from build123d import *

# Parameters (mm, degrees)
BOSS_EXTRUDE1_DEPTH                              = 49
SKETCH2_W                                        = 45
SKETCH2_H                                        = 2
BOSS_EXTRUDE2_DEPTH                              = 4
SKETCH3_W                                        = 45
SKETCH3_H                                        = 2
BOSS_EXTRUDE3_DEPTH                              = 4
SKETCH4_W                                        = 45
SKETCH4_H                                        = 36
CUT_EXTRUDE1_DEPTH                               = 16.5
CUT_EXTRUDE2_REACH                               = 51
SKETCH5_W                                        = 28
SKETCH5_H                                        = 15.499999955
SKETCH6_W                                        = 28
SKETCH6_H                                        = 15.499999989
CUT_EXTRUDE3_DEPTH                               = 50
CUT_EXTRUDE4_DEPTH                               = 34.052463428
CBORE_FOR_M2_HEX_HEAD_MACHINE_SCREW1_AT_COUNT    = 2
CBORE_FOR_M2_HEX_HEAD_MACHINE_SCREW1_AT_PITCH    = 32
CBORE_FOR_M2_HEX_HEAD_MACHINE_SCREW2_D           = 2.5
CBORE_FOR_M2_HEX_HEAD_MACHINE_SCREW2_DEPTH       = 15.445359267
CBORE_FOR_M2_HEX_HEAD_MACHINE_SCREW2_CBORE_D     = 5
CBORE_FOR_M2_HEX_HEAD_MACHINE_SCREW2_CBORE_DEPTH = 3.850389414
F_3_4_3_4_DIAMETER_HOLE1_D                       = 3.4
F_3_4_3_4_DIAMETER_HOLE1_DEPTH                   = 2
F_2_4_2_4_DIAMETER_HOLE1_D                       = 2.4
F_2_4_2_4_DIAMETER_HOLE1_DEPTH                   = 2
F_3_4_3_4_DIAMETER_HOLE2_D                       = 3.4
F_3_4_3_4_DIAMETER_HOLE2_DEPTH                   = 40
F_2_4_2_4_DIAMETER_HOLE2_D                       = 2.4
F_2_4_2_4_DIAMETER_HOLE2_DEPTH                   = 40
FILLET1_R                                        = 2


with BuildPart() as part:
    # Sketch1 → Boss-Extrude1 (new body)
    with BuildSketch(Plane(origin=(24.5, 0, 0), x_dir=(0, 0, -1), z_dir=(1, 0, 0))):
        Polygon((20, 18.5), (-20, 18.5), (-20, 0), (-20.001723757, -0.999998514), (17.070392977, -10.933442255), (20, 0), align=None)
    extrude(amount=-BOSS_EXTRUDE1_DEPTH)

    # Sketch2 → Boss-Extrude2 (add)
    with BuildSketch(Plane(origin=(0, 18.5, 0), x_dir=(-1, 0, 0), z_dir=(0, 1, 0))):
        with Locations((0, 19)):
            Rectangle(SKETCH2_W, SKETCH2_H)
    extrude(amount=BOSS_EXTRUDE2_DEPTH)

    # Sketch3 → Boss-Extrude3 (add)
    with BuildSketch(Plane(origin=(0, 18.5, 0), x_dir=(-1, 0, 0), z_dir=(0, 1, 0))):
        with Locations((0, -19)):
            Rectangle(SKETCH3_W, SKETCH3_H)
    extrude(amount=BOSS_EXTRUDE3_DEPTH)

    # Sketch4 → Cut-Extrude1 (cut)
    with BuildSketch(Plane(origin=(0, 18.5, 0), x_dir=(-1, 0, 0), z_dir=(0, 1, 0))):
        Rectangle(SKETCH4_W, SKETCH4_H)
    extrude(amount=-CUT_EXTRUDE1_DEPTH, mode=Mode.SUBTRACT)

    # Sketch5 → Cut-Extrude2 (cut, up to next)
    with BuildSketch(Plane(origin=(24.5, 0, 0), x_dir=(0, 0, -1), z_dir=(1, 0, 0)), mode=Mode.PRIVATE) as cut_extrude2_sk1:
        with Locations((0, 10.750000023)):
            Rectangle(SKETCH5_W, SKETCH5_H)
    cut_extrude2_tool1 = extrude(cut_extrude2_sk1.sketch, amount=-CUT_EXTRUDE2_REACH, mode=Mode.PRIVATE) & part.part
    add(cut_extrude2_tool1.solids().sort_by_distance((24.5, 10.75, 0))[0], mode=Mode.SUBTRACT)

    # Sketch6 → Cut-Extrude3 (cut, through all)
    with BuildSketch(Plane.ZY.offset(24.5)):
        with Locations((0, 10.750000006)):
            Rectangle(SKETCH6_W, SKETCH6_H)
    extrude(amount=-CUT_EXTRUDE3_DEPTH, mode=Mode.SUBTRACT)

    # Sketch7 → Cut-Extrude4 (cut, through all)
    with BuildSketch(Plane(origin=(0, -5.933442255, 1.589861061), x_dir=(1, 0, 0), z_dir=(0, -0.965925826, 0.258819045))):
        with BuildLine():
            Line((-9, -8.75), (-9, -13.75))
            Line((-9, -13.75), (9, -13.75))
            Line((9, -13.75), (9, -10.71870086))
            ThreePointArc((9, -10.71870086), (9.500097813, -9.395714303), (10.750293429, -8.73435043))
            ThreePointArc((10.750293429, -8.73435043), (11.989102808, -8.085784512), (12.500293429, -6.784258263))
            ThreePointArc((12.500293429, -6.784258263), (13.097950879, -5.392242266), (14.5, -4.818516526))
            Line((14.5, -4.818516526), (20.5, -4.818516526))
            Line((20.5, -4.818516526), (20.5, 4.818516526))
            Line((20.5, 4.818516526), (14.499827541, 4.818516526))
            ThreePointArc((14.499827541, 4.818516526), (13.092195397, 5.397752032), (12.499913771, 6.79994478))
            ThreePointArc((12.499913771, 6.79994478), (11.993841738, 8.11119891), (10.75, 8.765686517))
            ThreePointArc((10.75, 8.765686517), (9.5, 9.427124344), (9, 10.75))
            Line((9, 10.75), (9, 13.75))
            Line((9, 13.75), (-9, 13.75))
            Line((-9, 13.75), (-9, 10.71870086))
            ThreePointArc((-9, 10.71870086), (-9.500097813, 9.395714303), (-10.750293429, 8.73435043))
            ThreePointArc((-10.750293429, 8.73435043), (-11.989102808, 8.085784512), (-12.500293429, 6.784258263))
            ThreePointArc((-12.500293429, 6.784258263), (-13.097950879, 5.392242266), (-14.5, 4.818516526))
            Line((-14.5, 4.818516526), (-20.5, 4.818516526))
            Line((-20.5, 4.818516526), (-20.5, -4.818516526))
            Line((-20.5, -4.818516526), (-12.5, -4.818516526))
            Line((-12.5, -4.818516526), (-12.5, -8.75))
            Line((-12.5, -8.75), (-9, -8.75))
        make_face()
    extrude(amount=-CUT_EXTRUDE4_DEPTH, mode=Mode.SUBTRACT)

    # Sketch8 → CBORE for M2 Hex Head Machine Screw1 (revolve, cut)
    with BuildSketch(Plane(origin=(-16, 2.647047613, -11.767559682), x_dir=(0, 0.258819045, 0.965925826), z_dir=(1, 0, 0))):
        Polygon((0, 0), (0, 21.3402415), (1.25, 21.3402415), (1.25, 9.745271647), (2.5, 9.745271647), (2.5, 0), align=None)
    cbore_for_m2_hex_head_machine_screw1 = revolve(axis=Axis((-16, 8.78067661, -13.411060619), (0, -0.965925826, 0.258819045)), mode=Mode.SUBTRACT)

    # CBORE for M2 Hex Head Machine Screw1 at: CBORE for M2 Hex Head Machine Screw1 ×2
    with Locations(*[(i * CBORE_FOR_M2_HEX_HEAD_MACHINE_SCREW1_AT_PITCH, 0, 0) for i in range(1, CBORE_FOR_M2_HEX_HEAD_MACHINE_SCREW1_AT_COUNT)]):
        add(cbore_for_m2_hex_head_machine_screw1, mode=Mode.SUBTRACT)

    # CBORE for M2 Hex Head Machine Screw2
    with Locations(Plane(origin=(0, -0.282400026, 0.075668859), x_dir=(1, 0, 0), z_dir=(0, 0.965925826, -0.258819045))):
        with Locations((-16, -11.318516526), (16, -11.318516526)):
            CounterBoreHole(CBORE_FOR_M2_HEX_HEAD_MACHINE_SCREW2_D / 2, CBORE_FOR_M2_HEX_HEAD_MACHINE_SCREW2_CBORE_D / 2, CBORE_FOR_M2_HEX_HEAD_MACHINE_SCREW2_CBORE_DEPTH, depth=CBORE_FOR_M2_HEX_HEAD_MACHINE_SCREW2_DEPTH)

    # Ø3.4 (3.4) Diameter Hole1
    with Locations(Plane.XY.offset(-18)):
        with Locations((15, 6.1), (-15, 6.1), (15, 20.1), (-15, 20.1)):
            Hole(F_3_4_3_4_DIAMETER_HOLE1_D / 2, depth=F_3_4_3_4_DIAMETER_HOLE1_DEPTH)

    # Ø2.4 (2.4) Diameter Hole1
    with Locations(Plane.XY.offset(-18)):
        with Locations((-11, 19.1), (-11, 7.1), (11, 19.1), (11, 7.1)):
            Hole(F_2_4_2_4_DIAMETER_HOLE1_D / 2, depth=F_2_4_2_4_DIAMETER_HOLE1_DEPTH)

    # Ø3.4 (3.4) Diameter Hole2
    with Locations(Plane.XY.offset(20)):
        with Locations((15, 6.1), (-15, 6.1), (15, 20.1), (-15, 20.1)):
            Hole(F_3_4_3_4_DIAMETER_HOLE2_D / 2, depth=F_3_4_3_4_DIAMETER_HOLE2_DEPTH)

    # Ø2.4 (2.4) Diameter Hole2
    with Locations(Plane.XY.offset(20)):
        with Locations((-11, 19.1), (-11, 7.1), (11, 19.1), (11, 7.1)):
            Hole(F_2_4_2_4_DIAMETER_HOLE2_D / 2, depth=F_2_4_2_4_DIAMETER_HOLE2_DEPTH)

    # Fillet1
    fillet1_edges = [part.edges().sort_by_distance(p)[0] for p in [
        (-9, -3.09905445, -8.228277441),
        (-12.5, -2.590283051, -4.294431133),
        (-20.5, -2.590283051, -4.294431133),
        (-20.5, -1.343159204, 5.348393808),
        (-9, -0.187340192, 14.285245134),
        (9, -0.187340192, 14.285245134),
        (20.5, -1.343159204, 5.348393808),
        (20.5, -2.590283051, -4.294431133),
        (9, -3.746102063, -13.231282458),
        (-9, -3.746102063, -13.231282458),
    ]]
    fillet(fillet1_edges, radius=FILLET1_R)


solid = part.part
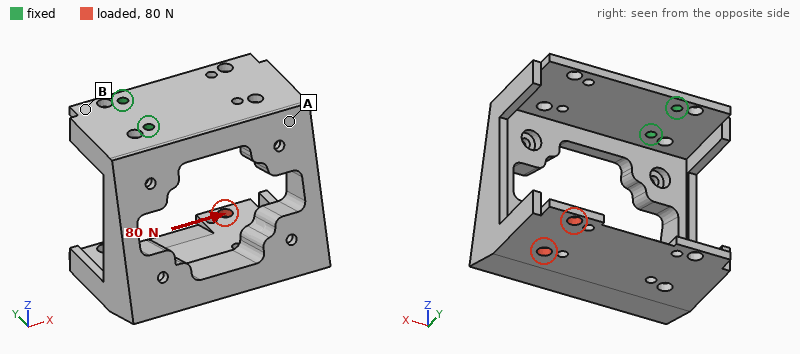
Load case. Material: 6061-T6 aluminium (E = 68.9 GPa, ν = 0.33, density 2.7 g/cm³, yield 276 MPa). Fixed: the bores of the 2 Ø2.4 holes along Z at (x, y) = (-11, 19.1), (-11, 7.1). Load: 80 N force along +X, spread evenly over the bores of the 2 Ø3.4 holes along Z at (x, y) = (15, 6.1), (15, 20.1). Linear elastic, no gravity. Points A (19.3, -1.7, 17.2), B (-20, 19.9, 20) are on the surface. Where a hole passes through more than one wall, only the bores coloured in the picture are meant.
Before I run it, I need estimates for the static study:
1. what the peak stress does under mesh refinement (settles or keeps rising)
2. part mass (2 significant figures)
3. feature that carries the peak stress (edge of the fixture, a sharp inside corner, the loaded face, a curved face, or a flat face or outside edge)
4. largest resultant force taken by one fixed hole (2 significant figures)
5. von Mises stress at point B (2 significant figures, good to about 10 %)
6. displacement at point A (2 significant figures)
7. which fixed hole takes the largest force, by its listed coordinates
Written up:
keeps rising
35 g
edge of the fixture
49 N
25 MPa
0.30 mm
(-11, 19.1)
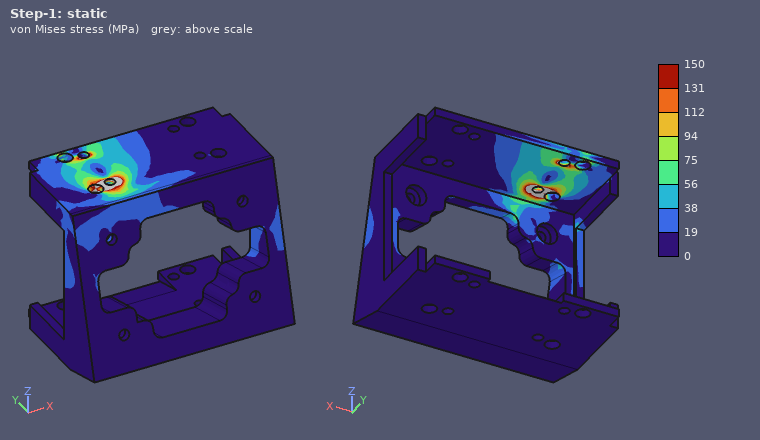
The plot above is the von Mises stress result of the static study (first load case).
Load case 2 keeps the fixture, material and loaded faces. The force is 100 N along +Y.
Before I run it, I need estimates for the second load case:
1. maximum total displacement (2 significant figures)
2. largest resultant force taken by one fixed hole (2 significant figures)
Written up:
0.76 mm
290 N
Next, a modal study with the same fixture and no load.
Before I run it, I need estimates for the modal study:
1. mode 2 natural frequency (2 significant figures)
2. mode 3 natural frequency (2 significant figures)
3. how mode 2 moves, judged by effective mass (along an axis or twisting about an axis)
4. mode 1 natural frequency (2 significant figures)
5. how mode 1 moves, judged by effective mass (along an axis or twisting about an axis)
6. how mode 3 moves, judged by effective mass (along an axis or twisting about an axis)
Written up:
490 Hz
2000 Hz
along Y
450 Hz
along X
along Z
